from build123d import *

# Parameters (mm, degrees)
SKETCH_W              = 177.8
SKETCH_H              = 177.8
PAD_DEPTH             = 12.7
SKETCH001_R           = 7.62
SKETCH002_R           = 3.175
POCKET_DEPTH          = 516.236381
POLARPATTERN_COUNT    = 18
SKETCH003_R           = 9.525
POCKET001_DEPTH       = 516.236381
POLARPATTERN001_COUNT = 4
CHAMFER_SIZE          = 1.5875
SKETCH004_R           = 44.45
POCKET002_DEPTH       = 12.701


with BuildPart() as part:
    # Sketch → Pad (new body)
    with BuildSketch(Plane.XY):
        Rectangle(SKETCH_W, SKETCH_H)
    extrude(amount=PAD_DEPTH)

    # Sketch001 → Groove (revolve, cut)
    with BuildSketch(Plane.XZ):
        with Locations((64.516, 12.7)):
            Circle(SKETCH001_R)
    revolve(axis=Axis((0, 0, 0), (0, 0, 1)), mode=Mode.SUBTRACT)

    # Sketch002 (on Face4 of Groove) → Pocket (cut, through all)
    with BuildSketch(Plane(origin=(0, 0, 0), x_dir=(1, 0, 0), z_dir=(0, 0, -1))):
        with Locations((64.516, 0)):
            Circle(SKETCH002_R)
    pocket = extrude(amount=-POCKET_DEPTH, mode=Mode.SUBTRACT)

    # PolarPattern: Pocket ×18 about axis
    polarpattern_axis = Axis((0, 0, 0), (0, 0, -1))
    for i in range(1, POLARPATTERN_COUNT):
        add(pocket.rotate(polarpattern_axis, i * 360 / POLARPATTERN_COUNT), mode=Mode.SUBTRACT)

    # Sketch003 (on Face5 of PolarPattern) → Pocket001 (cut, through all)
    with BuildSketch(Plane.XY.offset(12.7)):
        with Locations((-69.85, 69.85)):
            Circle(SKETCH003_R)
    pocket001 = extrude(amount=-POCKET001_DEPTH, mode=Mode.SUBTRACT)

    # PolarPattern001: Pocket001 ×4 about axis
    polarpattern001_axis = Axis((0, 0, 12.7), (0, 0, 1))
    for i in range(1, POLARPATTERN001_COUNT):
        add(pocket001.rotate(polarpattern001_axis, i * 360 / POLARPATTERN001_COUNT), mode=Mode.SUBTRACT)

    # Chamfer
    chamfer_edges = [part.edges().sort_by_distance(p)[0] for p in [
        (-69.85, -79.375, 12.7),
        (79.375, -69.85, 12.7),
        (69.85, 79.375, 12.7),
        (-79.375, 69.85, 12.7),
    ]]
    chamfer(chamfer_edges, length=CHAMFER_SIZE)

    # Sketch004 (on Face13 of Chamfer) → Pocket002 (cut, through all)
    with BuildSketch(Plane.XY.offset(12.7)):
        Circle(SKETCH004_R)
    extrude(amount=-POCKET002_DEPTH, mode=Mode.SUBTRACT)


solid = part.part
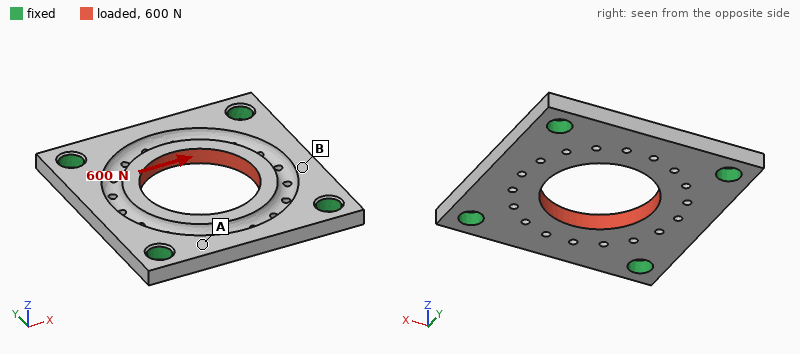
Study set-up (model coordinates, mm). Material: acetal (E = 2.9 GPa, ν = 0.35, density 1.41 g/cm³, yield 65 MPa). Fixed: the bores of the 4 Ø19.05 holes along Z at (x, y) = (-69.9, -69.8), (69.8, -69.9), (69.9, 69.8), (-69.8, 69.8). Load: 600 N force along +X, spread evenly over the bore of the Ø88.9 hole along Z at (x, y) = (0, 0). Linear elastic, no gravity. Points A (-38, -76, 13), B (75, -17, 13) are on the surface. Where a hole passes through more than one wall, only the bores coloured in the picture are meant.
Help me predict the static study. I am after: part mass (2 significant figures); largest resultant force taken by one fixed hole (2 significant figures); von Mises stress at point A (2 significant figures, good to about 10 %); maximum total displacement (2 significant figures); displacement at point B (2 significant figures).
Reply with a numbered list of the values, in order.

1. 380 g
2. 150 N
3. 0.20 MPa
4. 21 µm
5. 9.8 µm
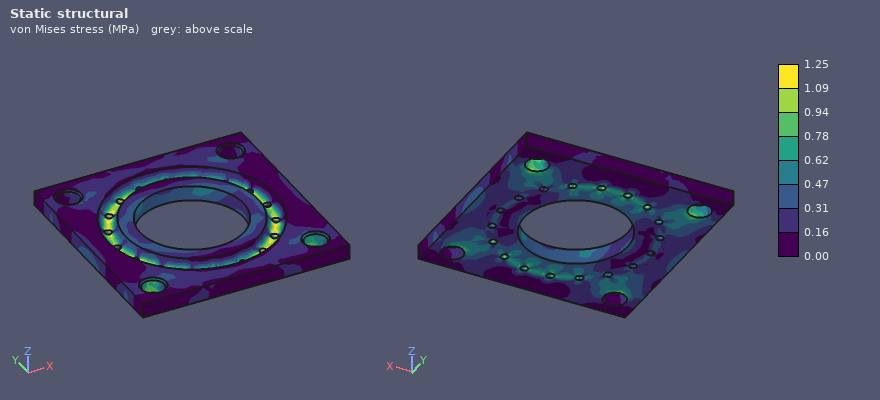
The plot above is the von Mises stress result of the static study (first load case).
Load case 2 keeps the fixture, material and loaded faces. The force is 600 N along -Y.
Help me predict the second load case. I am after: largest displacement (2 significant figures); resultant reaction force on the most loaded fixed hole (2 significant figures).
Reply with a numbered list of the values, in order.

1. 21 µm
2. 150 N
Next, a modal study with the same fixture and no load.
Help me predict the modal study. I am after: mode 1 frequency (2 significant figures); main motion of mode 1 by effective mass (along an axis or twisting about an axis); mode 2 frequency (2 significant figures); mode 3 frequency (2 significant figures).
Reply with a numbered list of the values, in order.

1. 940 Hz
2. along Z
3. 1100 Hz
4. 1100 Hz
